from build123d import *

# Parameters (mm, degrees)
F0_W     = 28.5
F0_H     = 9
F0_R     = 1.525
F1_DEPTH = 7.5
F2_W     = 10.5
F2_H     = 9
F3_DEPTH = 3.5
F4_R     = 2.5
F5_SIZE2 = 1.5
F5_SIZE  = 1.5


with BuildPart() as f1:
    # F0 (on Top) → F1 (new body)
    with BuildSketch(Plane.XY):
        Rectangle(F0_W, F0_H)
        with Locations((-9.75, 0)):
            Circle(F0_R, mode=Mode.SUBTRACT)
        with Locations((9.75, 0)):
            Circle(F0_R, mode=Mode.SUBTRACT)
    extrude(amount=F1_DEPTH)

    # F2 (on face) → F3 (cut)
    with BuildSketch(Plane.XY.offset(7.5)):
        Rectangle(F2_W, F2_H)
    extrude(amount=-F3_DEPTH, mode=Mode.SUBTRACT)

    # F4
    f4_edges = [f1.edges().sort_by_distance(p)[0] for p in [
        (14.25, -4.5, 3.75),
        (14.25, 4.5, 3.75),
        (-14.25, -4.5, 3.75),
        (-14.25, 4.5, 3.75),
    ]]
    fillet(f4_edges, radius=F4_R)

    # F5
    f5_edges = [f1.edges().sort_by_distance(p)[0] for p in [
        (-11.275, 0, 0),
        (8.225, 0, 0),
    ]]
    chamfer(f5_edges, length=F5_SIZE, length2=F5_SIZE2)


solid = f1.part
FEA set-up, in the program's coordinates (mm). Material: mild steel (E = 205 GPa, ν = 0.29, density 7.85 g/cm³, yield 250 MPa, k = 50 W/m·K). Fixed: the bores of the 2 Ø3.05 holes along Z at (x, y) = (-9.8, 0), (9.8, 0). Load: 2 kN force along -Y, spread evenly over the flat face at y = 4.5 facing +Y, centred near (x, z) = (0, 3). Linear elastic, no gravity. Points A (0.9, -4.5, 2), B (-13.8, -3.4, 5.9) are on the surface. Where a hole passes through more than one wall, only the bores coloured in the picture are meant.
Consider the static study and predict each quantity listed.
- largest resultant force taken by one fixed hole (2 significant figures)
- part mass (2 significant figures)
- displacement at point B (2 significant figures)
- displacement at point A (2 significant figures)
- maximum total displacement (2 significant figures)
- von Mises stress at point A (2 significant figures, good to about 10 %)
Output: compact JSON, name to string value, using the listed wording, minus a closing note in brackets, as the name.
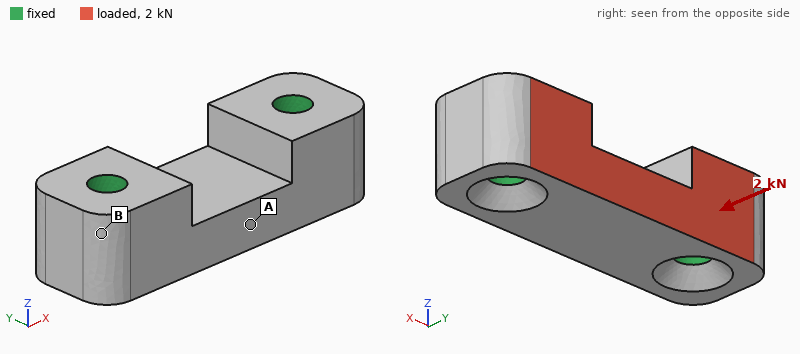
{"largest resultant force taken by one fixed hole": "1.0 kN", "part mass": "11 g", "displacement at point B": "0.34 µm", "displacement at point A": "1.6 µm", "maximum total displacement": "2.2 µm", "von Mises stress at point A": "25 MPa"}
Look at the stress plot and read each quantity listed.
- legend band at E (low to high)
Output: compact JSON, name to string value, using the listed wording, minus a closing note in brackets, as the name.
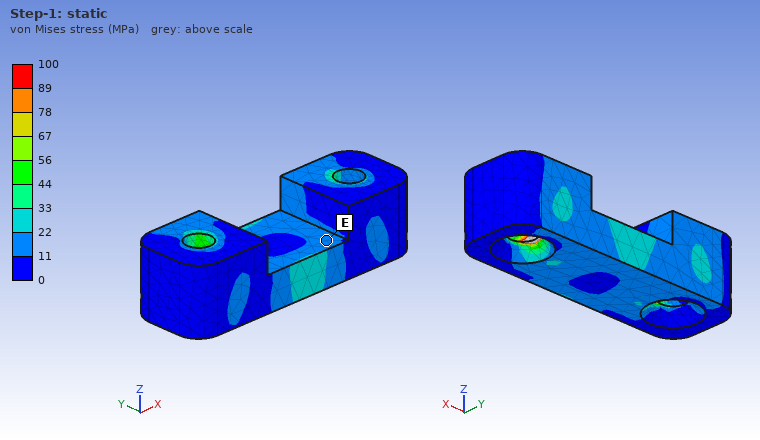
{"legend band at E": "11 to 22 MPa"}
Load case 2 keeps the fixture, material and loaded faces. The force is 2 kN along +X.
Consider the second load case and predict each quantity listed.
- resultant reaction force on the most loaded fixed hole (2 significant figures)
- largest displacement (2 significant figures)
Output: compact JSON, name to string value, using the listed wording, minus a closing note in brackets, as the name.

{"resultant reaction force on the most loaded fixed hole": "1.0 kN", "largest displacement": "1.5 µm"}
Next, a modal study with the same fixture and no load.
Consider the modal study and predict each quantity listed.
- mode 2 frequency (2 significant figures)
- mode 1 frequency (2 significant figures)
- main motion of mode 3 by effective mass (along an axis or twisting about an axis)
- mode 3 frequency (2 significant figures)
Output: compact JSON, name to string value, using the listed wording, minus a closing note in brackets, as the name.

{"mode 2 frequency": "62 kHz", "mode 1 frequency": "59 kHz", "main motion of mode 3 by effective mass": "twisting about X", "mode 3 frequency": "80 kHz"}
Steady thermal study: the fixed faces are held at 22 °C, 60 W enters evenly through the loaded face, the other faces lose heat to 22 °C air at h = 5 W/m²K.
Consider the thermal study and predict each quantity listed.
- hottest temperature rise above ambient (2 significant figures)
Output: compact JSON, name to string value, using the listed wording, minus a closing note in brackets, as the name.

{"hottest temperature rise above ambient": "68 K"}
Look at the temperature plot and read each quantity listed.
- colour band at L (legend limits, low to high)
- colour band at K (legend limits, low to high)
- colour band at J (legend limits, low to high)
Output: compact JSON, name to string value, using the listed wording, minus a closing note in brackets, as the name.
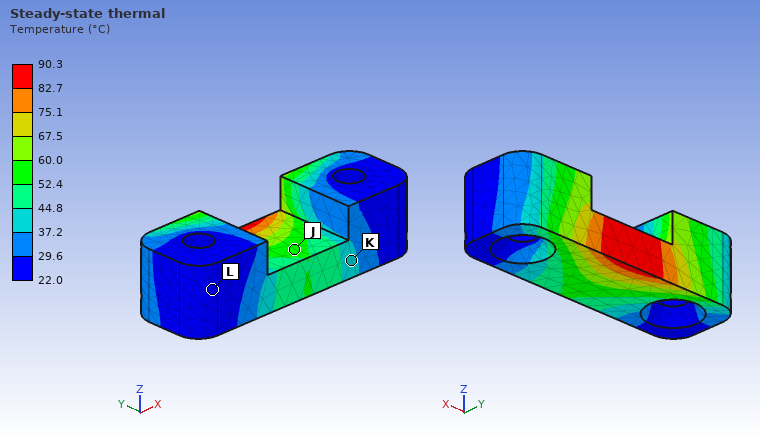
{"colour band at L": "22.0 to 29.6 °C", "colour band at K": "37.2 to 44.8 °C", "colour band at J": "52.4 to 60.0 °C"}
